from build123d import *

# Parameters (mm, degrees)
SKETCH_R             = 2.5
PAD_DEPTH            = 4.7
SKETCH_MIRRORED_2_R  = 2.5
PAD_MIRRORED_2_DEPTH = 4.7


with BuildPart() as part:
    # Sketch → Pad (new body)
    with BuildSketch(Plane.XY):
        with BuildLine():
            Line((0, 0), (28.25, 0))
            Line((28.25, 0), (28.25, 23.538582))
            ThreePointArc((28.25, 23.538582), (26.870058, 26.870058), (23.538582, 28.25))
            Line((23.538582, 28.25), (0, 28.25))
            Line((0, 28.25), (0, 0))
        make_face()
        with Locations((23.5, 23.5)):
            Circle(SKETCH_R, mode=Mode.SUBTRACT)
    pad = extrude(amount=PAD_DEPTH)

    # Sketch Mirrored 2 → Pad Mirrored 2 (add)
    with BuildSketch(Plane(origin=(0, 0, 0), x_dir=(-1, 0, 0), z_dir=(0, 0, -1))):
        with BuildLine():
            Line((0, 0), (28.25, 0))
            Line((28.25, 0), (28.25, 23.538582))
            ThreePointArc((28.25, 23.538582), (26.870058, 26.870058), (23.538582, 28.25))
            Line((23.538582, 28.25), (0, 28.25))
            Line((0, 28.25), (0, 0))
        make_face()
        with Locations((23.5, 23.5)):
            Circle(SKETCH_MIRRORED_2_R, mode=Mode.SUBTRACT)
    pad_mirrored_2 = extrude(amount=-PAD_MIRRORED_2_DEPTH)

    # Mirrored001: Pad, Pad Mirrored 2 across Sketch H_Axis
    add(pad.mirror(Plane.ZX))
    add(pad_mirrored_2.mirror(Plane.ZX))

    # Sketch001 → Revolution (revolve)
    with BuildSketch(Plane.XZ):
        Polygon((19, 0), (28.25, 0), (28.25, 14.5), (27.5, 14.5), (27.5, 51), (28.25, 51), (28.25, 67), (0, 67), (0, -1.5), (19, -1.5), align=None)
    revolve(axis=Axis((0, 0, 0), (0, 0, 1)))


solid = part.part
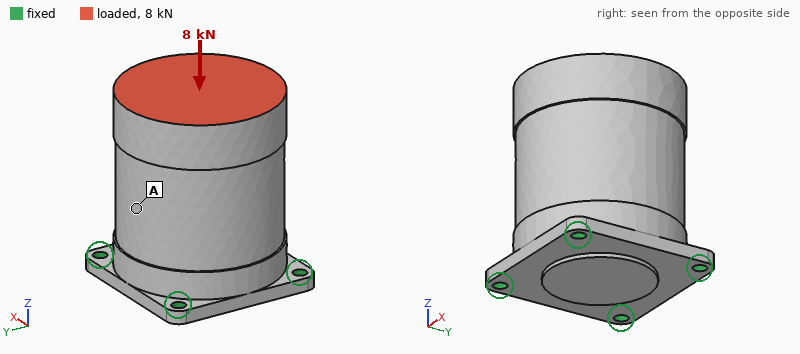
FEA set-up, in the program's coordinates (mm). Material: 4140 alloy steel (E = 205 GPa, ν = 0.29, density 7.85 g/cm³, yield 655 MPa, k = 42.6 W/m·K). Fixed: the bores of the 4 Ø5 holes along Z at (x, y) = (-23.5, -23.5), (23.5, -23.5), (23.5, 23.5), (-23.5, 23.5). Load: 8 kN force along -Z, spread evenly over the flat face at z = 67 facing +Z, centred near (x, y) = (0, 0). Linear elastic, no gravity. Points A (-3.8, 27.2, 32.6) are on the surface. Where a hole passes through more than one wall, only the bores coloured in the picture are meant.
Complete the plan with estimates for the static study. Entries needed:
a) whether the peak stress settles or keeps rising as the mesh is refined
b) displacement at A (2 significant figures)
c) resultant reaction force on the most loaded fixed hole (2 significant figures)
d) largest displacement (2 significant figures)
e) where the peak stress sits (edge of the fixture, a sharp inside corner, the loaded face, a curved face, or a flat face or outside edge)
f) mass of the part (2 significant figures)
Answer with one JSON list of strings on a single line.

["keeps rising", "5.2 µm", "2.2 kN", "5.8 µm", "edge of the fixture", "1.3 kg"]
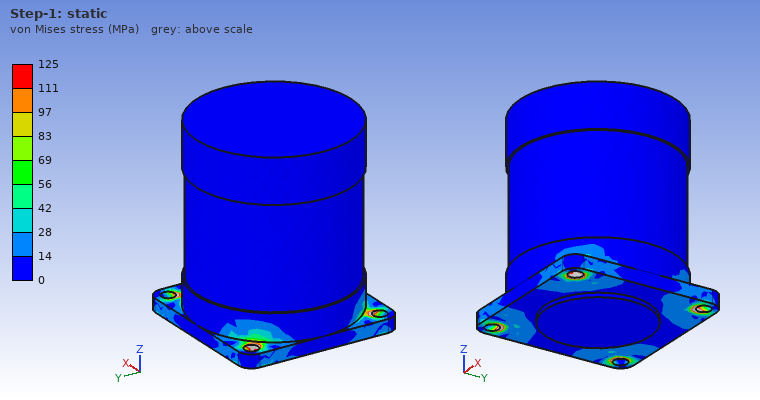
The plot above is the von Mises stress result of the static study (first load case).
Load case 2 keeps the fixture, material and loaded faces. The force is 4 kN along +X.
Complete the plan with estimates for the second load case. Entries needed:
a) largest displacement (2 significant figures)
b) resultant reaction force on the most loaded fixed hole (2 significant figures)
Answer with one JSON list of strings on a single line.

["29 µm", "3.3 kN"]
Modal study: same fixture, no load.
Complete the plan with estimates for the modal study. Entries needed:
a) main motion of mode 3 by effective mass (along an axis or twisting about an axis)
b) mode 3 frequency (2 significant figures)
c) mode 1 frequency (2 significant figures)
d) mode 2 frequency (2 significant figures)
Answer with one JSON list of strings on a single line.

["along Z", "5500 Hz", "2900 Hz", "2900 Hz"]
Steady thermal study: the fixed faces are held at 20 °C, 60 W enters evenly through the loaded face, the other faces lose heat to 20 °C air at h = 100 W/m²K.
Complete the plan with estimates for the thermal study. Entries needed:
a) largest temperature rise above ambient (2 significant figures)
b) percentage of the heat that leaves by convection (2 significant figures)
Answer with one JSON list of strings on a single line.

["42 K", "59 %"]
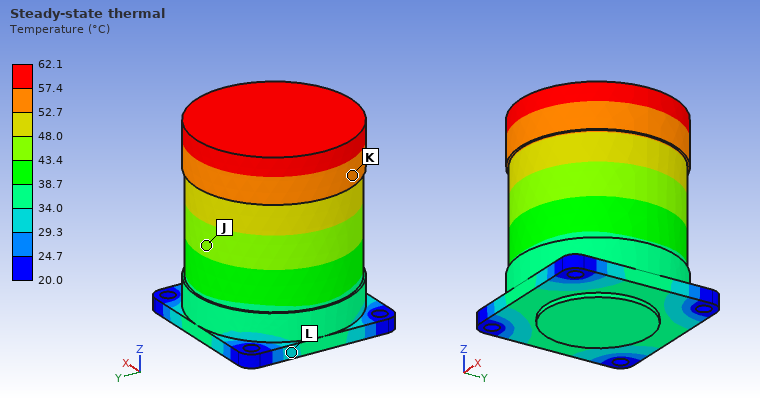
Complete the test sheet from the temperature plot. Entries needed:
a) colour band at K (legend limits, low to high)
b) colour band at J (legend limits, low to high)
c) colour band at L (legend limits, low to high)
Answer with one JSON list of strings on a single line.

["52.7 to 57.4 °C", "43.4 to 48.0 °C", "29.3 to 34.0 °C"]
